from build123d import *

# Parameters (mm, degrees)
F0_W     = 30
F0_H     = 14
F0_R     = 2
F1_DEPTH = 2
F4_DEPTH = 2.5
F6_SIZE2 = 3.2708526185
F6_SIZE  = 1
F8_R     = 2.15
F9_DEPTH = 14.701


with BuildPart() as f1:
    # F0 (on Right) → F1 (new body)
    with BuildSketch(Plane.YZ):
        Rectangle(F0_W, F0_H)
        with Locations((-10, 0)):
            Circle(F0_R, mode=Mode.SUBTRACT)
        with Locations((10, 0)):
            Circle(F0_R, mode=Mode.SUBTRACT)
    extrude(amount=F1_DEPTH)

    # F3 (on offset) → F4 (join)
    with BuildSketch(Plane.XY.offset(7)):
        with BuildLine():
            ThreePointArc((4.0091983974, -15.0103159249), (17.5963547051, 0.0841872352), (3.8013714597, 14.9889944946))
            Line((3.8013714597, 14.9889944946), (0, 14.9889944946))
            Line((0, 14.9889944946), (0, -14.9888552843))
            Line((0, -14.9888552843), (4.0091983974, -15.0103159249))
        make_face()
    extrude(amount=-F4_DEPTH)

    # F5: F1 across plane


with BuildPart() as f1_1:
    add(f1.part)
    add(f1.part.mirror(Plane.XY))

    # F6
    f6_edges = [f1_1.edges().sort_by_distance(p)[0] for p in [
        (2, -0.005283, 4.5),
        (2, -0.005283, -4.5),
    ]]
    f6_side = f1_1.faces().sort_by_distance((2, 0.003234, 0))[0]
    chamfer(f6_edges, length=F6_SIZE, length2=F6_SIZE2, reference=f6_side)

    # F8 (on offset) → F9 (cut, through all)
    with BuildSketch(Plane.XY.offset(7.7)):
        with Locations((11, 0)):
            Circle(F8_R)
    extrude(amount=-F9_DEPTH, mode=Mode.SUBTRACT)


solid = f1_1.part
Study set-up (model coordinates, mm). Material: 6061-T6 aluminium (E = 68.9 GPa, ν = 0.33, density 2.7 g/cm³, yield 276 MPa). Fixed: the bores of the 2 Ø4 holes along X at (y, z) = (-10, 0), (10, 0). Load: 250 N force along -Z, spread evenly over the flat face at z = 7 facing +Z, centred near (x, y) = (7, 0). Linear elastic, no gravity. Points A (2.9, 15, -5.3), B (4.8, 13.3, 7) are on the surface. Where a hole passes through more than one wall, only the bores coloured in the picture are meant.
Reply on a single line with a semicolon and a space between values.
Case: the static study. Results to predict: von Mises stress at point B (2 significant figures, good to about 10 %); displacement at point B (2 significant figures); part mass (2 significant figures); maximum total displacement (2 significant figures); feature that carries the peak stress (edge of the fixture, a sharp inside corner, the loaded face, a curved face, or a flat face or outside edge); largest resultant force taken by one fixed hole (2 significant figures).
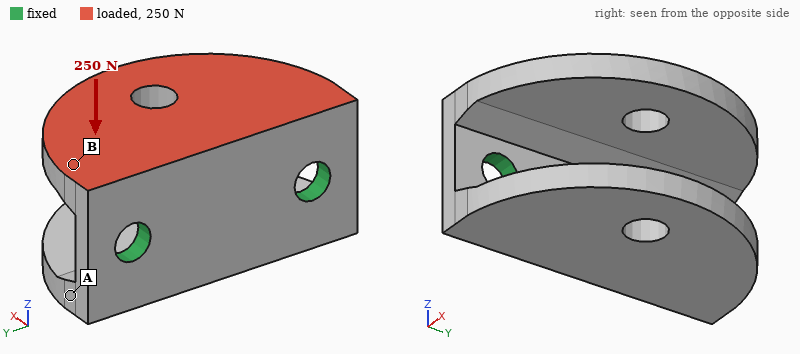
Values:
24 MPa; 23 µm; 7.2 g; 92 µm; a flat face or outside edge; 130 N
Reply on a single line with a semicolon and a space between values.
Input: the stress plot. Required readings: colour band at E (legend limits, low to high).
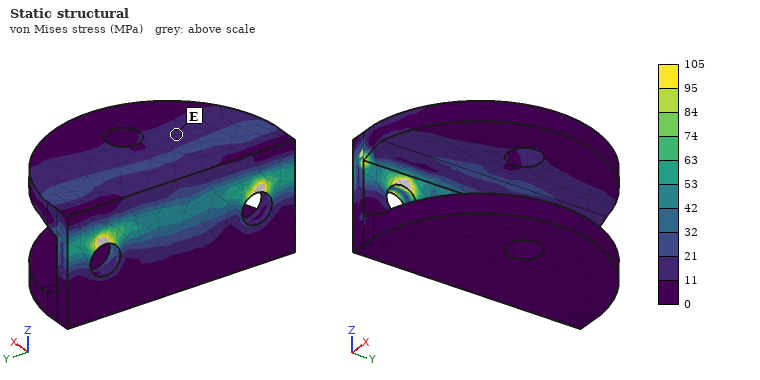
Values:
11 to 21 MPa
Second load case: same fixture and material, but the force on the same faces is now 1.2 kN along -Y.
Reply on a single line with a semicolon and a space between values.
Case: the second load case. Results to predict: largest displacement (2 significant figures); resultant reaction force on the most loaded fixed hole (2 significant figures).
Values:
24 µm; 780 N
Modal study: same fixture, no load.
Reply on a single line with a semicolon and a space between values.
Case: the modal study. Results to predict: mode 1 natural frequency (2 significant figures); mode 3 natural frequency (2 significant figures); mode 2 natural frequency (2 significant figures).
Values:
6200 Hz; 14 kHz; 6400 Hz
